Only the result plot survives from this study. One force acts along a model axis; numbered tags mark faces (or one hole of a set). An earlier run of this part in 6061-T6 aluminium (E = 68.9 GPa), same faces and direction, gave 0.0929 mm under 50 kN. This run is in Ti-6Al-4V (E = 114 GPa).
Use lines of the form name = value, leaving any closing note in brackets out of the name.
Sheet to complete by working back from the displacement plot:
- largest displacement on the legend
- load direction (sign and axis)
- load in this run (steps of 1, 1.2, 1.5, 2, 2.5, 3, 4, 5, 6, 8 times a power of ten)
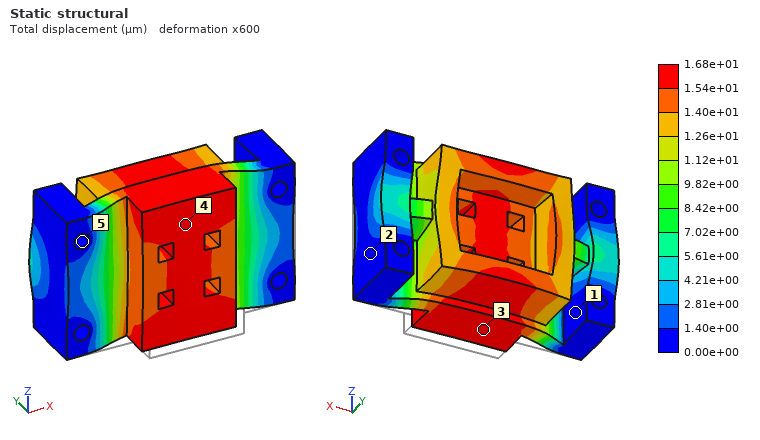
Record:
largest displacement on the legend = 1.68e+01 µm
load direction = +Y
load in this run = 15 kN
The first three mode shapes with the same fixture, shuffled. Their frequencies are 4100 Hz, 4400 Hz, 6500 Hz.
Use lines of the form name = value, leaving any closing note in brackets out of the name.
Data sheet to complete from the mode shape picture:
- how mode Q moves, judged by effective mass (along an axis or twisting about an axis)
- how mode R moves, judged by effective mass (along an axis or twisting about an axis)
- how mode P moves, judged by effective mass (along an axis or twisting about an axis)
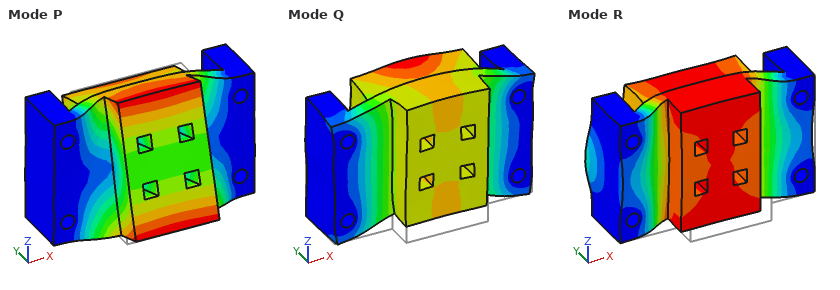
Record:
how mode Q moves, judged by effective mass = along Z
how mode R moves, judged by effective mass = along Y
how mode P moves, judged by effective mass = twisting about X
